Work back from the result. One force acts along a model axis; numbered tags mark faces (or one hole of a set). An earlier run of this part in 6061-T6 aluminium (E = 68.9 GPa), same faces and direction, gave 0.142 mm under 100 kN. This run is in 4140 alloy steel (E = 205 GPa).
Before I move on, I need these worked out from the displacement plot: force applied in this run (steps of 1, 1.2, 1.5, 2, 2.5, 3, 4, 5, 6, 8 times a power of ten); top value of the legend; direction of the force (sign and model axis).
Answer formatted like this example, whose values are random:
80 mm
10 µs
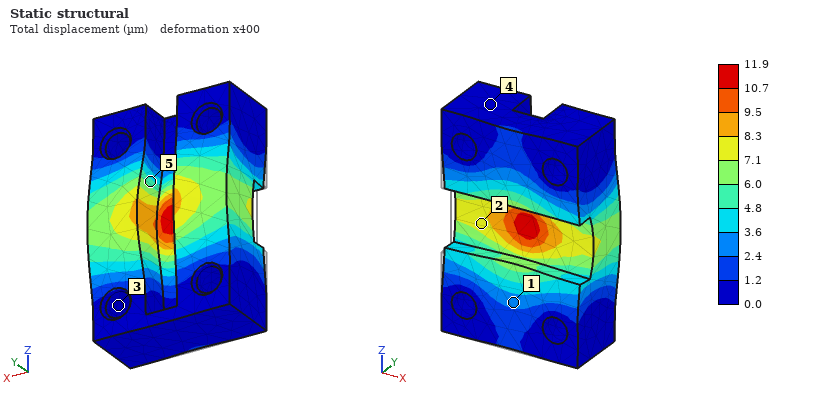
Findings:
25 kN
11.9 µm
+Y
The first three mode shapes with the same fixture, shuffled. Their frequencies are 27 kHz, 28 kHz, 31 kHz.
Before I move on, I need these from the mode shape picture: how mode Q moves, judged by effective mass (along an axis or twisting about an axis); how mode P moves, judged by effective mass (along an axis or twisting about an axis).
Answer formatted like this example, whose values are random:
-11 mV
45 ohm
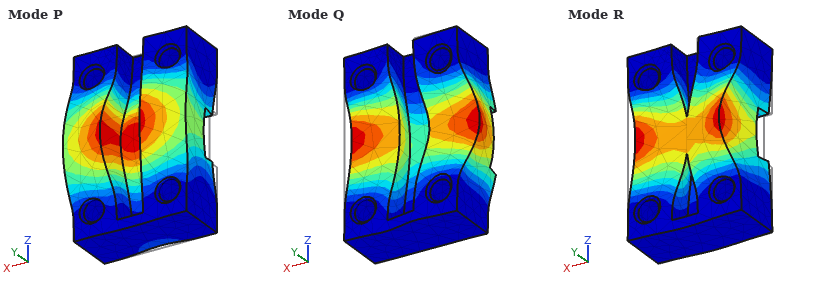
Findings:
along X
along Y
